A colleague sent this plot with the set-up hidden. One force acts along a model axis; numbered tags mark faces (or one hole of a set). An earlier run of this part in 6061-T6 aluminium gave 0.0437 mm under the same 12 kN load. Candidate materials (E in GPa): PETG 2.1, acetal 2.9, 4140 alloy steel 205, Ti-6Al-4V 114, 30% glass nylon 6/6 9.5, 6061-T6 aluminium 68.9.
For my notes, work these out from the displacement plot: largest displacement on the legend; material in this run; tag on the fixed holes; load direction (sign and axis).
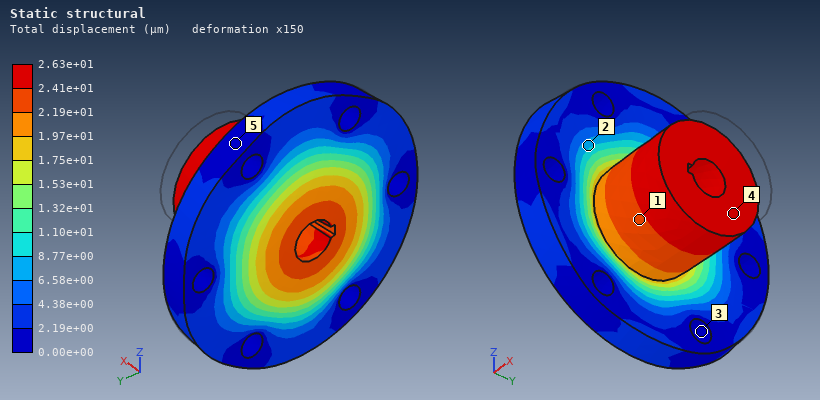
2.63e+01 µm
Ti-6Al-4V
3
-X
